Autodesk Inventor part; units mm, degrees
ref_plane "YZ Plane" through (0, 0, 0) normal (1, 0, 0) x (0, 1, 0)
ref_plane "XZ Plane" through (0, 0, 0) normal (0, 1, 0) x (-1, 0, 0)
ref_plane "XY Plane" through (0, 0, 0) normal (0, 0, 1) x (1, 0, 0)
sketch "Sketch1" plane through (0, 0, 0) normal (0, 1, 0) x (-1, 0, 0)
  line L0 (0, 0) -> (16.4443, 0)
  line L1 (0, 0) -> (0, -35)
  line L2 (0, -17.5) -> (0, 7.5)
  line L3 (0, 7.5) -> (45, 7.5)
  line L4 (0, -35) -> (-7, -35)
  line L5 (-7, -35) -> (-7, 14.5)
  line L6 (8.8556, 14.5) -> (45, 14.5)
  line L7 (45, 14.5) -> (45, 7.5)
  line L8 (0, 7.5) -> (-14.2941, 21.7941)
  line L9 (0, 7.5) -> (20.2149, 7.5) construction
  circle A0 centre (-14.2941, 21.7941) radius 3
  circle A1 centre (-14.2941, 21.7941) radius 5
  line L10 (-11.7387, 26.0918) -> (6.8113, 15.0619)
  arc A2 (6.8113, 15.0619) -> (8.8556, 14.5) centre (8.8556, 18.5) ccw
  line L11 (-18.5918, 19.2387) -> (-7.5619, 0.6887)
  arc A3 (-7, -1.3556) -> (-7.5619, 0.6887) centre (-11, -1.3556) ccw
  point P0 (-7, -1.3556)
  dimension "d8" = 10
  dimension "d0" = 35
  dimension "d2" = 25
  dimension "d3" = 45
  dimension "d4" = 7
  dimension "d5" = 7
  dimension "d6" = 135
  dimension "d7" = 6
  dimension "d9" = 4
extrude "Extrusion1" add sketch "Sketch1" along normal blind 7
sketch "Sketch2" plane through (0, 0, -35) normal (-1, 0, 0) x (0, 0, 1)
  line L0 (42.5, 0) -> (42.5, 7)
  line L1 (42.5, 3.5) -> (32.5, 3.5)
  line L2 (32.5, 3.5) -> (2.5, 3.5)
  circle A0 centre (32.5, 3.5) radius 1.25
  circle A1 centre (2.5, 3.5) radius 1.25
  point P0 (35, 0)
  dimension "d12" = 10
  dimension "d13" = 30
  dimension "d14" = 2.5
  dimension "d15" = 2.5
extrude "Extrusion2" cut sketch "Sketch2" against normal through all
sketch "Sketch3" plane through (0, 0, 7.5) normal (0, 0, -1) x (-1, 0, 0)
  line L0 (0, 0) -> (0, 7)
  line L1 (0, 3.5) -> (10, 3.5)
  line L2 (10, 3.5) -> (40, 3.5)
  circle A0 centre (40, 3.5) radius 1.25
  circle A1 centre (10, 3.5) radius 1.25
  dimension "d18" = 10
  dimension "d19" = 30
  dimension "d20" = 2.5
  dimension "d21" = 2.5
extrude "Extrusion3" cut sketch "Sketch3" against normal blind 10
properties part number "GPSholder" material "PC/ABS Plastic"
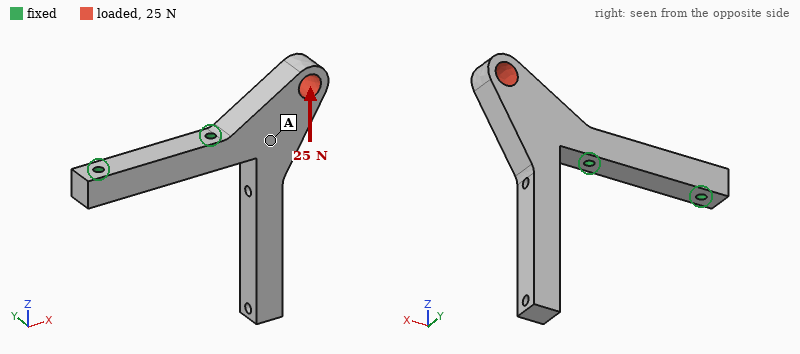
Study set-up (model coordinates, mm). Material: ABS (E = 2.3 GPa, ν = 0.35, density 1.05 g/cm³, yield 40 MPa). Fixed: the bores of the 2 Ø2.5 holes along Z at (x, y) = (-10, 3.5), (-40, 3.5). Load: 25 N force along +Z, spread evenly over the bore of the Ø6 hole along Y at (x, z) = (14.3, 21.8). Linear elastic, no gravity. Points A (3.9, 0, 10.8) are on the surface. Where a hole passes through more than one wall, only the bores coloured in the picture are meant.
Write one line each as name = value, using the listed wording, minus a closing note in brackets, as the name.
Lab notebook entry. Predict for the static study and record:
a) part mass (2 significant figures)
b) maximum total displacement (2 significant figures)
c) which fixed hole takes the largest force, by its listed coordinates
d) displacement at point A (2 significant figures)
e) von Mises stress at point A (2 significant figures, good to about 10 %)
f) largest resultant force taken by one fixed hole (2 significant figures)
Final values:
part mass = 6.4 g
maximum total displacement = 0.40 mm
which fixed hole takes the largest force, by its listed coordinates = (-10, 3.5)
displacement at point A = 0.085 mm
von Mises stress at point A = 1.2 MPa
largest resultant force taken by one fixed hole = 27 N
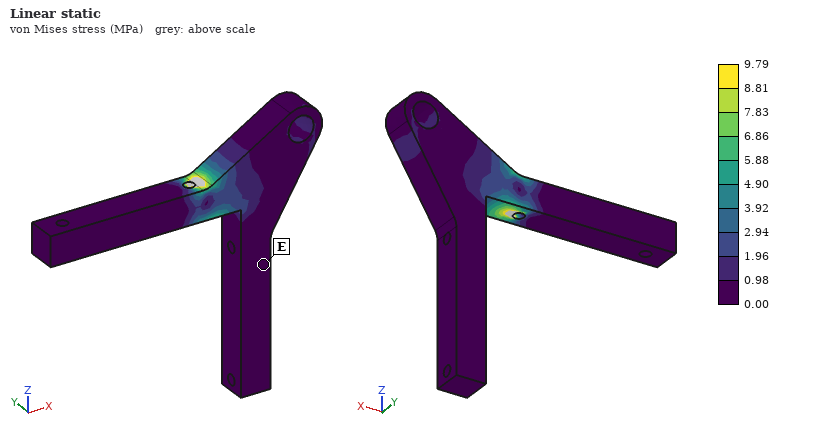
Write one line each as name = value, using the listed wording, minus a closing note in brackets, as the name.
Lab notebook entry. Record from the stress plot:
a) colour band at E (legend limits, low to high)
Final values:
colour band at E = 0.00 to 0.98 MPa
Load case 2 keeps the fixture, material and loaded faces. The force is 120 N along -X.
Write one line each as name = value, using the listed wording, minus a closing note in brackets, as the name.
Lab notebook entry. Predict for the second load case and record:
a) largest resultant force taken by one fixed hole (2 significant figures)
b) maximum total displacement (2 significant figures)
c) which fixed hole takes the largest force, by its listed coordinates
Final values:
largest resultant force taken by one fixed hole = 120 N
maximum total displacement = 0.94 mm
which fixed hole takes the largest force, by its listed coordinates = (-10, 3.5)
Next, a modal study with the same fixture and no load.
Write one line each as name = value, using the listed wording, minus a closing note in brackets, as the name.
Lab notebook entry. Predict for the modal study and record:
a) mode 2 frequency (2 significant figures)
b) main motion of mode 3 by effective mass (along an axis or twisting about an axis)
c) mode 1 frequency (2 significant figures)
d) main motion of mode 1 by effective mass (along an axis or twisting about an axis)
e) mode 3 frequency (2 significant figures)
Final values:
mode 2 frequency = 650 Hz
main motion of mode 3 by effective mass = along Y
mode 1 frequency = 550 Hz
main motion of mode 1 by effective mass = along Y
mode 3 frequency = 1300 Hz
